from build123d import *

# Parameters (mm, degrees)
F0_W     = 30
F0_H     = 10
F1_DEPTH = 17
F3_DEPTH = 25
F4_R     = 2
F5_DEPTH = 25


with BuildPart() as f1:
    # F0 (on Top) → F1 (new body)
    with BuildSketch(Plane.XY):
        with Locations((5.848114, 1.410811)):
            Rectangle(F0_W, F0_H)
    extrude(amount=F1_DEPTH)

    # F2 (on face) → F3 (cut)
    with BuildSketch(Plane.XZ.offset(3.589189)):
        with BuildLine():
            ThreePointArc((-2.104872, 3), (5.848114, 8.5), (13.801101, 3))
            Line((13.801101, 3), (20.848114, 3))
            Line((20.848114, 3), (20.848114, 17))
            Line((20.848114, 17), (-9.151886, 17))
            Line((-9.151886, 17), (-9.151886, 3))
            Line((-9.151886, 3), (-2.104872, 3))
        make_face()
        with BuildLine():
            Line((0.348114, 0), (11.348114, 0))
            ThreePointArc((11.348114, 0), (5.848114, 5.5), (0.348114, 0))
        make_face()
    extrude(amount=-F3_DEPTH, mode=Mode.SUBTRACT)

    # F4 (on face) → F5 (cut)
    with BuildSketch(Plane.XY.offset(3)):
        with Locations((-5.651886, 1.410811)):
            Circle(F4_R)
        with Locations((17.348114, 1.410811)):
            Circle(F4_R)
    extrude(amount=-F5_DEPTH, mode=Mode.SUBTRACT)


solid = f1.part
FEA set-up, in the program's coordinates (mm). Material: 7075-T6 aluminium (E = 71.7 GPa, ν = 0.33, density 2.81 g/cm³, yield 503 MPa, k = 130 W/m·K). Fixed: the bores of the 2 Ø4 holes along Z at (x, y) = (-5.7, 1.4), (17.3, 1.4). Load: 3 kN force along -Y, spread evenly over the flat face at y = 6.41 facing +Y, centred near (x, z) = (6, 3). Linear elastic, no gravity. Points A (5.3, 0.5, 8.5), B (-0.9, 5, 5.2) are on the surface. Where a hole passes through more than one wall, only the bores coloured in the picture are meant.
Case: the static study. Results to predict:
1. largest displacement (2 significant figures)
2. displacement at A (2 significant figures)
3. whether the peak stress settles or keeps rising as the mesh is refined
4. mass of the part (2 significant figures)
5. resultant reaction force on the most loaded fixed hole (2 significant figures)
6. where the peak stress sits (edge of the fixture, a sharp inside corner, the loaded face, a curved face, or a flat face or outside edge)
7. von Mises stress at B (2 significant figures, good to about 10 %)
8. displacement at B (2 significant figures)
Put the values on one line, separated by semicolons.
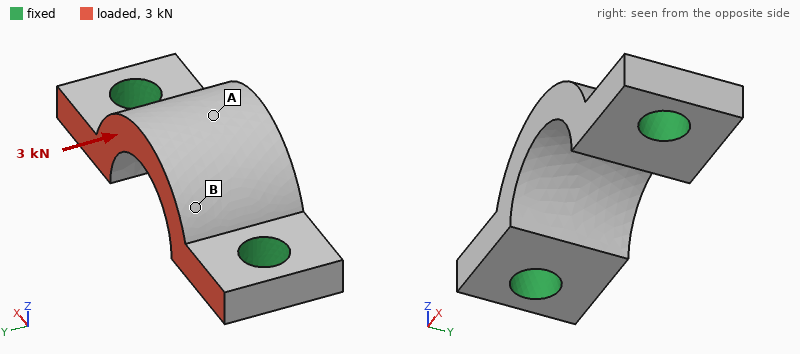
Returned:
53 µm; 44 µm; keeps rising; 2.8 g; 1.5 kN; edge of the fixture; 66 MPa; 28 µm
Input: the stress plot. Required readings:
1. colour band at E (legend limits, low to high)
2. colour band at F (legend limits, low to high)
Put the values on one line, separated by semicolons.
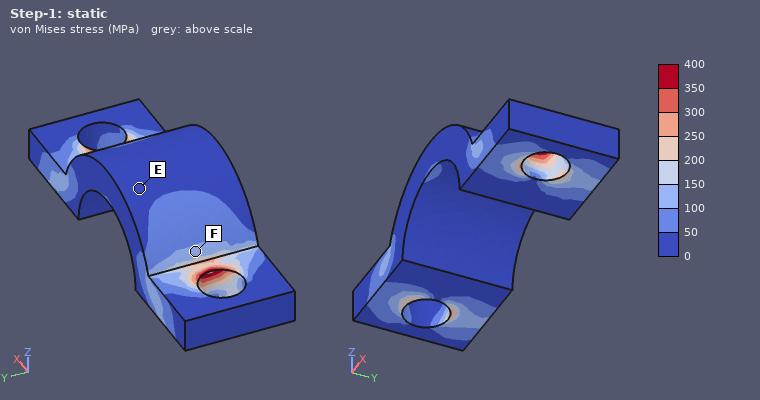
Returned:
0 to 50 MPa; 100 to 150 MPa
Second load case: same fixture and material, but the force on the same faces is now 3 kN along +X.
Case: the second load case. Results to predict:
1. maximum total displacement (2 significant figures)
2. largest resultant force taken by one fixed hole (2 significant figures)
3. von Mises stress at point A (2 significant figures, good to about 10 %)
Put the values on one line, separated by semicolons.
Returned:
24 µm; 1.6 kN; 36 MPa
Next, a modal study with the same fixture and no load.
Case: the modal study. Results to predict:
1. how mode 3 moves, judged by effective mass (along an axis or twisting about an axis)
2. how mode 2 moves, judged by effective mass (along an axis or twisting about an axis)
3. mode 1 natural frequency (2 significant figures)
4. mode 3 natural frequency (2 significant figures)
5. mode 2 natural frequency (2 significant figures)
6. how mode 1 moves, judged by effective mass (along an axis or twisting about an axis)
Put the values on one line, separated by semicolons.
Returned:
along X; along Z; 26 kHz; 54 kHz; 48 kHz; along Y
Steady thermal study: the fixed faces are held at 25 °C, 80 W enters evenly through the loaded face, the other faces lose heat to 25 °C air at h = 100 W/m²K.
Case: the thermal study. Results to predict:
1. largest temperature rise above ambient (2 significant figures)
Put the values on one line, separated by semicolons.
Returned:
67 K
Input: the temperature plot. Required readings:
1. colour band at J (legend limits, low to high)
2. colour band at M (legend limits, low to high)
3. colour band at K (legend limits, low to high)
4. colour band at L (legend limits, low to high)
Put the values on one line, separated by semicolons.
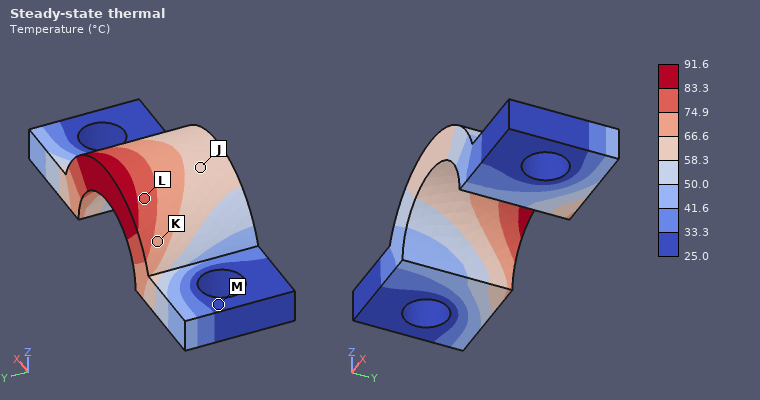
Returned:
58.3 to 66.6 °C; 25.0 to 33.3 °C; 66.6 to 74.9 °C; 74.9 to 83.3 °C
